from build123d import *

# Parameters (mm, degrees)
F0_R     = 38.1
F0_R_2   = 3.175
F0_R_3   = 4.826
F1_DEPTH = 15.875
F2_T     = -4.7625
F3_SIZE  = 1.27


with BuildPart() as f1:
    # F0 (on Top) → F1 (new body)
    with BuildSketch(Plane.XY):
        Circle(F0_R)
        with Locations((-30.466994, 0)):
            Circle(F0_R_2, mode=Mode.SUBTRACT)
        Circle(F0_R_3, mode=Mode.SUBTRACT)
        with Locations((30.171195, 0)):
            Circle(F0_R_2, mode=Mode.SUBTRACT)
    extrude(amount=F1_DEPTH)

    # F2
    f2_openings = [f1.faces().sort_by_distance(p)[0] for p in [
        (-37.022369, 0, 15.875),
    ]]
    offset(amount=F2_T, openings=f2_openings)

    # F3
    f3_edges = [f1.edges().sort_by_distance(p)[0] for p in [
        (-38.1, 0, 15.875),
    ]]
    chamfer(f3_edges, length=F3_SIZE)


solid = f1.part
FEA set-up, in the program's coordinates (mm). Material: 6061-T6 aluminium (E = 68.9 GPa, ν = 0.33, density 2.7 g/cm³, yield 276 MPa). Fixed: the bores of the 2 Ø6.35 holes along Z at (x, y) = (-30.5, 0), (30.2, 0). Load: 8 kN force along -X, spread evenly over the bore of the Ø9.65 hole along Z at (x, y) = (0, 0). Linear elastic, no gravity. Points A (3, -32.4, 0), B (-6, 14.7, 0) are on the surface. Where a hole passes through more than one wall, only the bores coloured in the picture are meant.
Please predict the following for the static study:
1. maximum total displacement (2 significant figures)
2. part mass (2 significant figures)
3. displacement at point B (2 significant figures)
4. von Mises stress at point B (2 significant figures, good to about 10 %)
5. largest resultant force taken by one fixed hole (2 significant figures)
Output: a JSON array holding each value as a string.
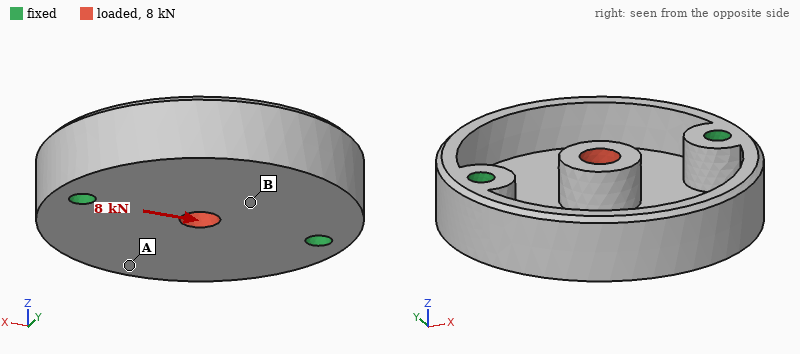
["70 µm", "100 g", "12 µm", "27 MPa", "4.1 kN"]
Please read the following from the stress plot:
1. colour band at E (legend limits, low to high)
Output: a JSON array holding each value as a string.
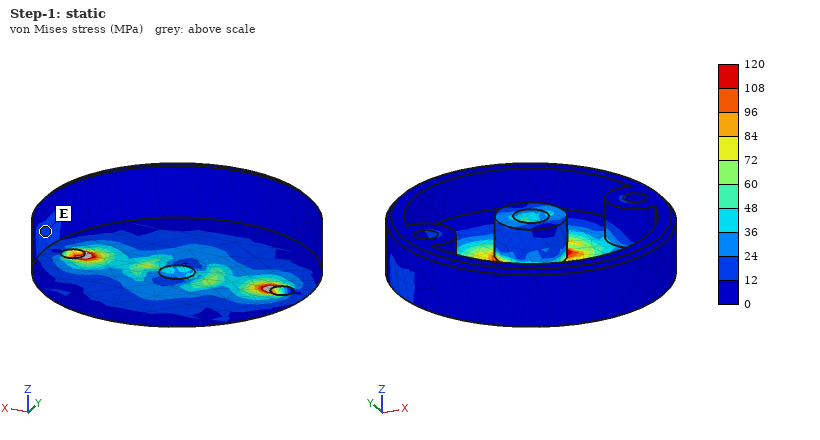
["12 to 24 MPa"]
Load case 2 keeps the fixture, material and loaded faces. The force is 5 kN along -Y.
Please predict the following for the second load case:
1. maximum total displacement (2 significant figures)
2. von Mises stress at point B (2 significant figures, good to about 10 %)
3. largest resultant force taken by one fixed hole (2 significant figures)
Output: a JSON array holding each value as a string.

["65 µm", "35 MPa", "2.5 kN"]
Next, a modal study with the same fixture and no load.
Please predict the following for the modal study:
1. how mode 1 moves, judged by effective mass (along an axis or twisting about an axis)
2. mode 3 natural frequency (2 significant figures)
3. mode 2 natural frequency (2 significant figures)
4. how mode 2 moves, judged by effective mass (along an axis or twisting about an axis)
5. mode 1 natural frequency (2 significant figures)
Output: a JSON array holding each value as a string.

["twisting about X", "9700 Hz", "5500 Hz", "along Z", "4900 Hz"]
